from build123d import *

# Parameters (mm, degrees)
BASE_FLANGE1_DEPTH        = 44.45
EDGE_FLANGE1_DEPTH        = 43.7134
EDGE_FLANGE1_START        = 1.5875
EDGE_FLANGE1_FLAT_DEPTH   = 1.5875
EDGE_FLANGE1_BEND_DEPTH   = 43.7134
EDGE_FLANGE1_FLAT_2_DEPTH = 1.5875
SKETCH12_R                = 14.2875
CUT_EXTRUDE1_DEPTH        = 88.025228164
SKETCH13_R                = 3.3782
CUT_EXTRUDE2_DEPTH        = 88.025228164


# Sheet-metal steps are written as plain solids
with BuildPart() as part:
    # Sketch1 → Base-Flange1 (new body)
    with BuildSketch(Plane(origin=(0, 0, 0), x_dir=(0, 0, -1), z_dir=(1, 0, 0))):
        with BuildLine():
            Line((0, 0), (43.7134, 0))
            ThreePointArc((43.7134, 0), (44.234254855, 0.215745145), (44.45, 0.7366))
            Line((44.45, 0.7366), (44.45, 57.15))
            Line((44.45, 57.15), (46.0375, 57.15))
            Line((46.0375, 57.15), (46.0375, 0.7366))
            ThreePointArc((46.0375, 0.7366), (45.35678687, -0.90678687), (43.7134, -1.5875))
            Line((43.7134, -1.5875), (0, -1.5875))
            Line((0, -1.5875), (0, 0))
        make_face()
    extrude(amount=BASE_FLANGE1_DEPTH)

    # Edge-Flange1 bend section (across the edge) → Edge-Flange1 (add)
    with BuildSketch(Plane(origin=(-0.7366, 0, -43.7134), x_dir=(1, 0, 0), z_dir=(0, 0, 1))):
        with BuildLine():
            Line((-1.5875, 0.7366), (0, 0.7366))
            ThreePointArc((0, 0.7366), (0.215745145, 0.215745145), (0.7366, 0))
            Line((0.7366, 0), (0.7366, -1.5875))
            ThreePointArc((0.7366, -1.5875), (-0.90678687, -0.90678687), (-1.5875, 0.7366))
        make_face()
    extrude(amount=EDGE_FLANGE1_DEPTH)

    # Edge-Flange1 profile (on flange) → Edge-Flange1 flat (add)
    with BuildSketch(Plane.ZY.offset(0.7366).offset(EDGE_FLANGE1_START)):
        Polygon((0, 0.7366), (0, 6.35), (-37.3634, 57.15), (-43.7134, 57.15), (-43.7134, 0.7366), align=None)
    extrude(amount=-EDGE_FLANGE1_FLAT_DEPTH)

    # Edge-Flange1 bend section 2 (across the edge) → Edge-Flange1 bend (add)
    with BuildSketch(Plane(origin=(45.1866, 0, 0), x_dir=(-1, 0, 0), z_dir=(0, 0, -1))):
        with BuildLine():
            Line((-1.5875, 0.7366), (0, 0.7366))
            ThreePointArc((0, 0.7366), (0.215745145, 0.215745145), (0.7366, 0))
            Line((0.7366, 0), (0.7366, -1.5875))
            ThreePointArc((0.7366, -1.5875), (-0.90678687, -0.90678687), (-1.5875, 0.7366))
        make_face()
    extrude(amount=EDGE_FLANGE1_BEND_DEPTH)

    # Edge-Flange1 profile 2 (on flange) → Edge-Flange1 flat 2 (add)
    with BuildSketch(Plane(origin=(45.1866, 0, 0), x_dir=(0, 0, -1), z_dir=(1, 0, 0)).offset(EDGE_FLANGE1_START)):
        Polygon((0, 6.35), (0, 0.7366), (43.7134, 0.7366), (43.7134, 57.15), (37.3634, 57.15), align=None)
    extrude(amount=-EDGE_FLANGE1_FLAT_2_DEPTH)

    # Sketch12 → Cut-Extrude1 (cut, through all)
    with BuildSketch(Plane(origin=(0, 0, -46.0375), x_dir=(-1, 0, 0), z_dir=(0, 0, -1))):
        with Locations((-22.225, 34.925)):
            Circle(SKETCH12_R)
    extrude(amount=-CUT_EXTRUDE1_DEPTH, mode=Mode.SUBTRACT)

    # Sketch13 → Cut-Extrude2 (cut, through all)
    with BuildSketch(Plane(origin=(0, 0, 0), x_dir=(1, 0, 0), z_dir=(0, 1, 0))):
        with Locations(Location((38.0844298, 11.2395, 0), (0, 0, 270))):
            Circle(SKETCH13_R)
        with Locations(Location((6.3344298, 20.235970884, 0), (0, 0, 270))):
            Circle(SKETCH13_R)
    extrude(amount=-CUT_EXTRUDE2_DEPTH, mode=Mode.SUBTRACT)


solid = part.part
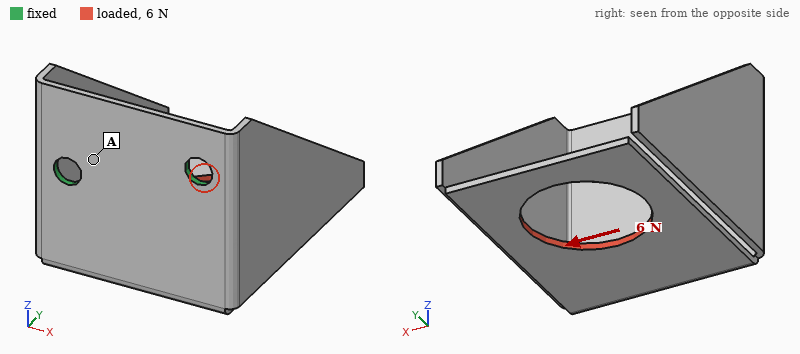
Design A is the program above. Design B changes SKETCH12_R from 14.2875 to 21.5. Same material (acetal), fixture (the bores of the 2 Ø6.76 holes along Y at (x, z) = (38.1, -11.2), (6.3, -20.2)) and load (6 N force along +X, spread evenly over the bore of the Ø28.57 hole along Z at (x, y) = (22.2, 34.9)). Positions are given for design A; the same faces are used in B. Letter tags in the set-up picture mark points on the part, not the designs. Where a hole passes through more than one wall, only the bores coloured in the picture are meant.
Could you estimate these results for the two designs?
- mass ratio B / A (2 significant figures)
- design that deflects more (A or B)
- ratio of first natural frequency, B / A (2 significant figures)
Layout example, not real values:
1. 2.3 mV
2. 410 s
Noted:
1. 0.89
2. B
3. 0.94
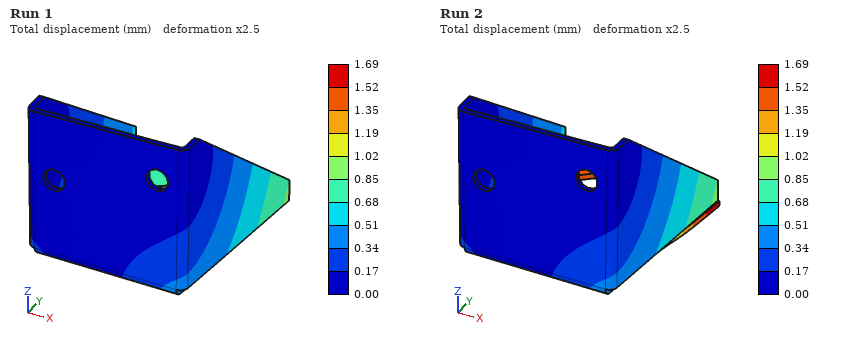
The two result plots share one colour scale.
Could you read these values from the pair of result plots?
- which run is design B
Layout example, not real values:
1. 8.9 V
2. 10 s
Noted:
1. Run 2
